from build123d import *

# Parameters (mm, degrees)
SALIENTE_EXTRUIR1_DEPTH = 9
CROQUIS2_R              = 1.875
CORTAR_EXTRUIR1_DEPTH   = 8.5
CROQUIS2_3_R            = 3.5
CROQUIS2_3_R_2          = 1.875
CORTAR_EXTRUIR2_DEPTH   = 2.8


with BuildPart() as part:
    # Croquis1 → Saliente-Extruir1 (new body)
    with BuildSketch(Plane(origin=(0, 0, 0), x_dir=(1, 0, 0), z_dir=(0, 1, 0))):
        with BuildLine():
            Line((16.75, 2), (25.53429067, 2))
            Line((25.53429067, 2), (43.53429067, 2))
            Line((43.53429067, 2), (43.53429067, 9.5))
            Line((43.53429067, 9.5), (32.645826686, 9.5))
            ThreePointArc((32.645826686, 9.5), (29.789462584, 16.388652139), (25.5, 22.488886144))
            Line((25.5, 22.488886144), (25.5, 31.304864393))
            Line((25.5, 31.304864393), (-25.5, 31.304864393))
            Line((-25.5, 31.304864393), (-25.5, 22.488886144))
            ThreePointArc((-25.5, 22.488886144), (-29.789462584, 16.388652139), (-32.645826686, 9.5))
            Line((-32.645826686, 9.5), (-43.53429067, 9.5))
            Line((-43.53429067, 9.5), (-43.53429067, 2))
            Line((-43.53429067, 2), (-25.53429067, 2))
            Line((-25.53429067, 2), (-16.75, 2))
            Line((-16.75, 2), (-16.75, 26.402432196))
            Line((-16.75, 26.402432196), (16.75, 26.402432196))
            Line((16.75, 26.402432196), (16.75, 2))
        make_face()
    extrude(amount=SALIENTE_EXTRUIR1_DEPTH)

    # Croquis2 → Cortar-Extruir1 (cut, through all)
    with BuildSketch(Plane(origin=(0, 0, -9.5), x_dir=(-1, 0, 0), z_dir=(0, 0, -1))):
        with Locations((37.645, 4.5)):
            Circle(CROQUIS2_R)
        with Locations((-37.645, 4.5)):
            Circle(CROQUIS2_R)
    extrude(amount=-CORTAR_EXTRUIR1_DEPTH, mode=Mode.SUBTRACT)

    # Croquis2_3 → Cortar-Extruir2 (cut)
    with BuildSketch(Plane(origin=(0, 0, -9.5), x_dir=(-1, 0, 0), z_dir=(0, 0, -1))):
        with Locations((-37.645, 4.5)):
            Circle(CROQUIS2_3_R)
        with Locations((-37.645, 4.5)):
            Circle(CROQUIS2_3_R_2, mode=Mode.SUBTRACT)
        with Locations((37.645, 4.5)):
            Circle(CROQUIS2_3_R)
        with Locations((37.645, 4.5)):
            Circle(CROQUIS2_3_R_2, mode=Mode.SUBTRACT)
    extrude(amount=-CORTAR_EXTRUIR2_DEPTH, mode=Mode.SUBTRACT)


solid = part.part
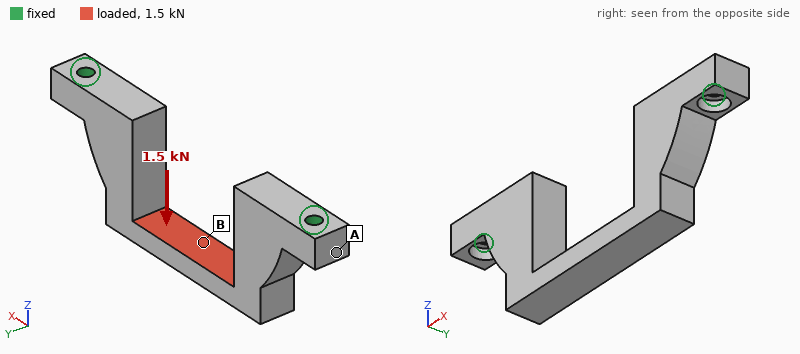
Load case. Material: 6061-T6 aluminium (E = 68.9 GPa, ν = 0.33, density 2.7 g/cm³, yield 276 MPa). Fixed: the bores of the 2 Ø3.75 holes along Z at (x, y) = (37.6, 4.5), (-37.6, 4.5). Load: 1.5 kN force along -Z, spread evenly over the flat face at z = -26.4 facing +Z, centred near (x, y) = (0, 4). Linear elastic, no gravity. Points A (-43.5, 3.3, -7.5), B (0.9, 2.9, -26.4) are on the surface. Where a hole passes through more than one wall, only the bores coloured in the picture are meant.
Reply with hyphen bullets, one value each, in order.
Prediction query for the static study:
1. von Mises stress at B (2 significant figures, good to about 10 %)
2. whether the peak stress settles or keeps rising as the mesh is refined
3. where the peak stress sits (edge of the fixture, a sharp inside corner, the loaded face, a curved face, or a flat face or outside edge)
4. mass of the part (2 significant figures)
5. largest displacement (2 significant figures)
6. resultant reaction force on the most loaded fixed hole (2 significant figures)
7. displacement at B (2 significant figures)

- 60 MPa
- keeps rising
- edge of the fixture
- 25 g
- 64 µm
- 1.0 kN
- 62 µm
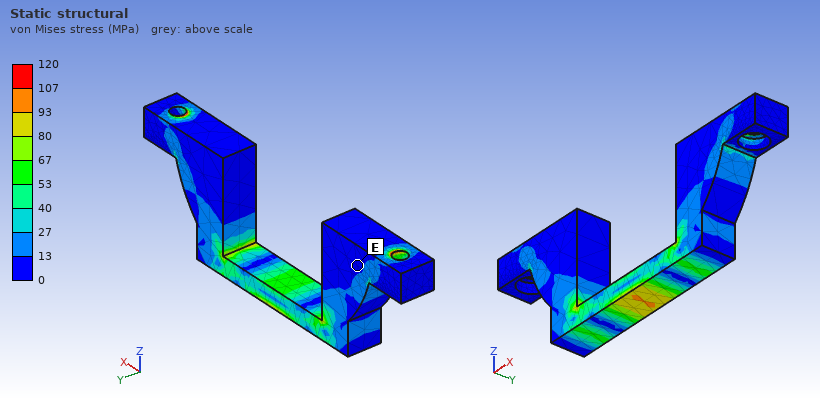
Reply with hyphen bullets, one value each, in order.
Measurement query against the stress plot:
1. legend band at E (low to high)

- 0 to 13 MPa
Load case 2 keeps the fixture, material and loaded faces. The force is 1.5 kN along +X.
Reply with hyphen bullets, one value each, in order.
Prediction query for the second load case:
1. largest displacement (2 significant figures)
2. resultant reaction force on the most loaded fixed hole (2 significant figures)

- 0.14 mm
- 800 N
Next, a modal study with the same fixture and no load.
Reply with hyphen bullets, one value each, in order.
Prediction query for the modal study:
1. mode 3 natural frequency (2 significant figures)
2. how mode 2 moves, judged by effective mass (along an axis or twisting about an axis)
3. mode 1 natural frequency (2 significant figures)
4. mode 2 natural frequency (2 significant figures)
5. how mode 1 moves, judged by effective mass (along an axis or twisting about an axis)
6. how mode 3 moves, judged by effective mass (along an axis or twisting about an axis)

- 6700 Hz
- along X
- 3200 Hz
- 5000 Hz
- along Y
- twisting about Z
